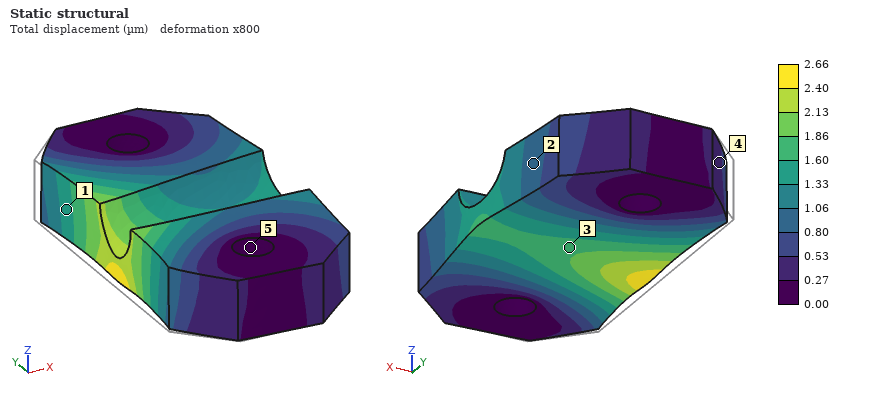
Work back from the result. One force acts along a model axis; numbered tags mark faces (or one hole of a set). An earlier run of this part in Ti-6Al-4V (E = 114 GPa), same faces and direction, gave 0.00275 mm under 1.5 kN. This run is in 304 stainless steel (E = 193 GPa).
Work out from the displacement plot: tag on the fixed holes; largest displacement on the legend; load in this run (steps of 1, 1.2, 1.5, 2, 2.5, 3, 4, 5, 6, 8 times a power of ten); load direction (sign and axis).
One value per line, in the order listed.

5
2.66 µm
2.5 kN
+X
